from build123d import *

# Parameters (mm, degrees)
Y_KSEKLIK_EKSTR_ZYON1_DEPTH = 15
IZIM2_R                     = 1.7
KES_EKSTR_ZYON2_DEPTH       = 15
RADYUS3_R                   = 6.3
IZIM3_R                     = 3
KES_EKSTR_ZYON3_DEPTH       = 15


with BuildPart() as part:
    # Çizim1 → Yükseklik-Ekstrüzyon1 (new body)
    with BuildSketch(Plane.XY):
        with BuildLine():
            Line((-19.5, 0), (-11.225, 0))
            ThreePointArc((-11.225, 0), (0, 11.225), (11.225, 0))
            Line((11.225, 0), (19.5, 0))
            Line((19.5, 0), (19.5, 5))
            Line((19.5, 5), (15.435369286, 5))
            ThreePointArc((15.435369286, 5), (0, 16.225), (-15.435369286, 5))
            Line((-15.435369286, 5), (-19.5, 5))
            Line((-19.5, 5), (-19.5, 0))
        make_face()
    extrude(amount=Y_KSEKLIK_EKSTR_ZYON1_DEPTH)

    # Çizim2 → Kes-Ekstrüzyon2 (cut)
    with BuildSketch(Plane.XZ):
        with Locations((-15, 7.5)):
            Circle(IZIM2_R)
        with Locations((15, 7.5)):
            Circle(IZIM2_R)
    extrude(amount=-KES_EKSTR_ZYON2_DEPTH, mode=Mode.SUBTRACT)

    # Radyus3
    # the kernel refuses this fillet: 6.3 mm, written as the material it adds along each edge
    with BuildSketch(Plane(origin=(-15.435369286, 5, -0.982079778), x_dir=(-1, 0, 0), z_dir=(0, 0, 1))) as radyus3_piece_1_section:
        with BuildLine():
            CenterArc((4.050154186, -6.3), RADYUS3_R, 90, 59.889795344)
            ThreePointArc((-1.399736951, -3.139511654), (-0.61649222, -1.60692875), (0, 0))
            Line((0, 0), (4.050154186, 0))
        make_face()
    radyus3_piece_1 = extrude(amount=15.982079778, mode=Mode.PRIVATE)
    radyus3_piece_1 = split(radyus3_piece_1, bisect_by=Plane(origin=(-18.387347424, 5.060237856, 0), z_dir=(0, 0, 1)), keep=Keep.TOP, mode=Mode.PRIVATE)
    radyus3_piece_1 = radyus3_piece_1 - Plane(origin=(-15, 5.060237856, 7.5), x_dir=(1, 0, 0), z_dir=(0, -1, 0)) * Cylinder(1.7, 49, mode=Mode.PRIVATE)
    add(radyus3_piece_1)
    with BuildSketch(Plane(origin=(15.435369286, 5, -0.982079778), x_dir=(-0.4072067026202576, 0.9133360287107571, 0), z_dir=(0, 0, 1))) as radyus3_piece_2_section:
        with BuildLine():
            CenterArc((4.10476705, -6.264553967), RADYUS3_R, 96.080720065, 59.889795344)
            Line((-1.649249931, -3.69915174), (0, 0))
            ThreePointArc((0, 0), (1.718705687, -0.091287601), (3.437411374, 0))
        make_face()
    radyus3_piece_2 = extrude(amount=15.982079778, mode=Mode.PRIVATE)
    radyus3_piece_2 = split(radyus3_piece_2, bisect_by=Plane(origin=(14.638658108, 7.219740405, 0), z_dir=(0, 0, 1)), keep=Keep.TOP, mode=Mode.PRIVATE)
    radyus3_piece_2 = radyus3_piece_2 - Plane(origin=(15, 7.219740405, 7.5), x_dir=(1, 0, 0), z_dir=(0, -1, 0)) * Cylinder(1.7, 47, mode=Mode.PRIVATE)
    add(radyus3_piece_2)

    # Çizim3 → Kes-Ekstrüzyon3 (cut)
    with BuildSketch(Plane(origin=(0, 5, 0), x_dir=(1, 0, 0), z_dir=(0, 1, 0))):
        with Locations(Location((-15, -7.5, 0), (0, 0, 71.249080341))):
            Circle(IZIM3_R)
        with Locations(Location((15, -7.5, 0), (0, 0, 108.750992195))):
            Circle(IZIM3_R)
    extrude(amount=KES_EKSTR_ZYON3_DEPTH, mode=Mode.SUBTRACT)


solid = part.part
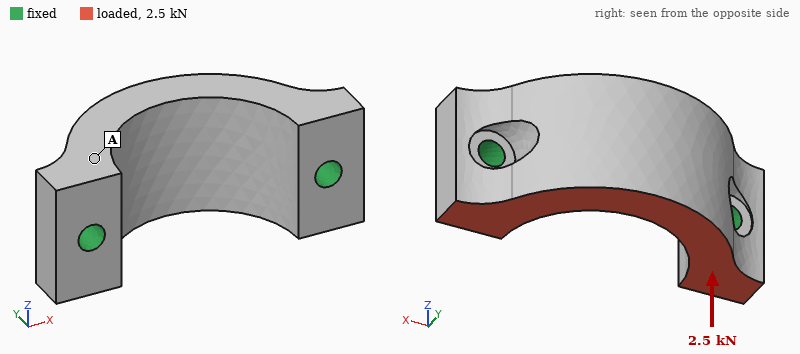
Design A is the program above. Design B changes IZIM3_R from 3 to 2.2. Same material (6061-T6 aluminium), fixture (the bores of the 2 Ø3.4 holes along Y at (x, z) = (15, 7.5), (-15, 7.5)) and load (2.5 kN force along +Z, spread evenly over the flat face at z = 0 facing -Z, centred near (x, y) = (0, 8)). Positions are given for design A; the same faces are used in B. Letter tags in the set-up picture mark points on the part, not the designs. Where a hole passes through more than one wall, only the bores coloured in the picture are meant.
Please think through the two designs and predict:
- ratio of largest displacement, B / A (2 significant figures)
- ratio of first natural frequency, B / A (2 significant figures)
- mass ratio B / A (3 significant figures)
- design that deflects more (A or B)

0.92
1.0
1.02
A
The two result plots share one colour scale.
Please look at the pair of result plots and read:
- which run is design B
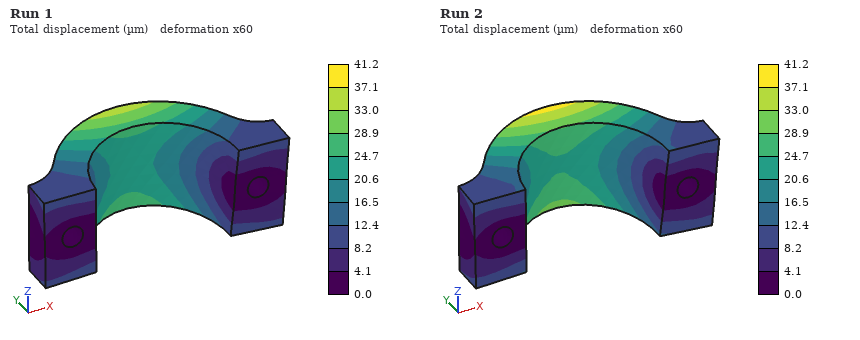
Run 1
